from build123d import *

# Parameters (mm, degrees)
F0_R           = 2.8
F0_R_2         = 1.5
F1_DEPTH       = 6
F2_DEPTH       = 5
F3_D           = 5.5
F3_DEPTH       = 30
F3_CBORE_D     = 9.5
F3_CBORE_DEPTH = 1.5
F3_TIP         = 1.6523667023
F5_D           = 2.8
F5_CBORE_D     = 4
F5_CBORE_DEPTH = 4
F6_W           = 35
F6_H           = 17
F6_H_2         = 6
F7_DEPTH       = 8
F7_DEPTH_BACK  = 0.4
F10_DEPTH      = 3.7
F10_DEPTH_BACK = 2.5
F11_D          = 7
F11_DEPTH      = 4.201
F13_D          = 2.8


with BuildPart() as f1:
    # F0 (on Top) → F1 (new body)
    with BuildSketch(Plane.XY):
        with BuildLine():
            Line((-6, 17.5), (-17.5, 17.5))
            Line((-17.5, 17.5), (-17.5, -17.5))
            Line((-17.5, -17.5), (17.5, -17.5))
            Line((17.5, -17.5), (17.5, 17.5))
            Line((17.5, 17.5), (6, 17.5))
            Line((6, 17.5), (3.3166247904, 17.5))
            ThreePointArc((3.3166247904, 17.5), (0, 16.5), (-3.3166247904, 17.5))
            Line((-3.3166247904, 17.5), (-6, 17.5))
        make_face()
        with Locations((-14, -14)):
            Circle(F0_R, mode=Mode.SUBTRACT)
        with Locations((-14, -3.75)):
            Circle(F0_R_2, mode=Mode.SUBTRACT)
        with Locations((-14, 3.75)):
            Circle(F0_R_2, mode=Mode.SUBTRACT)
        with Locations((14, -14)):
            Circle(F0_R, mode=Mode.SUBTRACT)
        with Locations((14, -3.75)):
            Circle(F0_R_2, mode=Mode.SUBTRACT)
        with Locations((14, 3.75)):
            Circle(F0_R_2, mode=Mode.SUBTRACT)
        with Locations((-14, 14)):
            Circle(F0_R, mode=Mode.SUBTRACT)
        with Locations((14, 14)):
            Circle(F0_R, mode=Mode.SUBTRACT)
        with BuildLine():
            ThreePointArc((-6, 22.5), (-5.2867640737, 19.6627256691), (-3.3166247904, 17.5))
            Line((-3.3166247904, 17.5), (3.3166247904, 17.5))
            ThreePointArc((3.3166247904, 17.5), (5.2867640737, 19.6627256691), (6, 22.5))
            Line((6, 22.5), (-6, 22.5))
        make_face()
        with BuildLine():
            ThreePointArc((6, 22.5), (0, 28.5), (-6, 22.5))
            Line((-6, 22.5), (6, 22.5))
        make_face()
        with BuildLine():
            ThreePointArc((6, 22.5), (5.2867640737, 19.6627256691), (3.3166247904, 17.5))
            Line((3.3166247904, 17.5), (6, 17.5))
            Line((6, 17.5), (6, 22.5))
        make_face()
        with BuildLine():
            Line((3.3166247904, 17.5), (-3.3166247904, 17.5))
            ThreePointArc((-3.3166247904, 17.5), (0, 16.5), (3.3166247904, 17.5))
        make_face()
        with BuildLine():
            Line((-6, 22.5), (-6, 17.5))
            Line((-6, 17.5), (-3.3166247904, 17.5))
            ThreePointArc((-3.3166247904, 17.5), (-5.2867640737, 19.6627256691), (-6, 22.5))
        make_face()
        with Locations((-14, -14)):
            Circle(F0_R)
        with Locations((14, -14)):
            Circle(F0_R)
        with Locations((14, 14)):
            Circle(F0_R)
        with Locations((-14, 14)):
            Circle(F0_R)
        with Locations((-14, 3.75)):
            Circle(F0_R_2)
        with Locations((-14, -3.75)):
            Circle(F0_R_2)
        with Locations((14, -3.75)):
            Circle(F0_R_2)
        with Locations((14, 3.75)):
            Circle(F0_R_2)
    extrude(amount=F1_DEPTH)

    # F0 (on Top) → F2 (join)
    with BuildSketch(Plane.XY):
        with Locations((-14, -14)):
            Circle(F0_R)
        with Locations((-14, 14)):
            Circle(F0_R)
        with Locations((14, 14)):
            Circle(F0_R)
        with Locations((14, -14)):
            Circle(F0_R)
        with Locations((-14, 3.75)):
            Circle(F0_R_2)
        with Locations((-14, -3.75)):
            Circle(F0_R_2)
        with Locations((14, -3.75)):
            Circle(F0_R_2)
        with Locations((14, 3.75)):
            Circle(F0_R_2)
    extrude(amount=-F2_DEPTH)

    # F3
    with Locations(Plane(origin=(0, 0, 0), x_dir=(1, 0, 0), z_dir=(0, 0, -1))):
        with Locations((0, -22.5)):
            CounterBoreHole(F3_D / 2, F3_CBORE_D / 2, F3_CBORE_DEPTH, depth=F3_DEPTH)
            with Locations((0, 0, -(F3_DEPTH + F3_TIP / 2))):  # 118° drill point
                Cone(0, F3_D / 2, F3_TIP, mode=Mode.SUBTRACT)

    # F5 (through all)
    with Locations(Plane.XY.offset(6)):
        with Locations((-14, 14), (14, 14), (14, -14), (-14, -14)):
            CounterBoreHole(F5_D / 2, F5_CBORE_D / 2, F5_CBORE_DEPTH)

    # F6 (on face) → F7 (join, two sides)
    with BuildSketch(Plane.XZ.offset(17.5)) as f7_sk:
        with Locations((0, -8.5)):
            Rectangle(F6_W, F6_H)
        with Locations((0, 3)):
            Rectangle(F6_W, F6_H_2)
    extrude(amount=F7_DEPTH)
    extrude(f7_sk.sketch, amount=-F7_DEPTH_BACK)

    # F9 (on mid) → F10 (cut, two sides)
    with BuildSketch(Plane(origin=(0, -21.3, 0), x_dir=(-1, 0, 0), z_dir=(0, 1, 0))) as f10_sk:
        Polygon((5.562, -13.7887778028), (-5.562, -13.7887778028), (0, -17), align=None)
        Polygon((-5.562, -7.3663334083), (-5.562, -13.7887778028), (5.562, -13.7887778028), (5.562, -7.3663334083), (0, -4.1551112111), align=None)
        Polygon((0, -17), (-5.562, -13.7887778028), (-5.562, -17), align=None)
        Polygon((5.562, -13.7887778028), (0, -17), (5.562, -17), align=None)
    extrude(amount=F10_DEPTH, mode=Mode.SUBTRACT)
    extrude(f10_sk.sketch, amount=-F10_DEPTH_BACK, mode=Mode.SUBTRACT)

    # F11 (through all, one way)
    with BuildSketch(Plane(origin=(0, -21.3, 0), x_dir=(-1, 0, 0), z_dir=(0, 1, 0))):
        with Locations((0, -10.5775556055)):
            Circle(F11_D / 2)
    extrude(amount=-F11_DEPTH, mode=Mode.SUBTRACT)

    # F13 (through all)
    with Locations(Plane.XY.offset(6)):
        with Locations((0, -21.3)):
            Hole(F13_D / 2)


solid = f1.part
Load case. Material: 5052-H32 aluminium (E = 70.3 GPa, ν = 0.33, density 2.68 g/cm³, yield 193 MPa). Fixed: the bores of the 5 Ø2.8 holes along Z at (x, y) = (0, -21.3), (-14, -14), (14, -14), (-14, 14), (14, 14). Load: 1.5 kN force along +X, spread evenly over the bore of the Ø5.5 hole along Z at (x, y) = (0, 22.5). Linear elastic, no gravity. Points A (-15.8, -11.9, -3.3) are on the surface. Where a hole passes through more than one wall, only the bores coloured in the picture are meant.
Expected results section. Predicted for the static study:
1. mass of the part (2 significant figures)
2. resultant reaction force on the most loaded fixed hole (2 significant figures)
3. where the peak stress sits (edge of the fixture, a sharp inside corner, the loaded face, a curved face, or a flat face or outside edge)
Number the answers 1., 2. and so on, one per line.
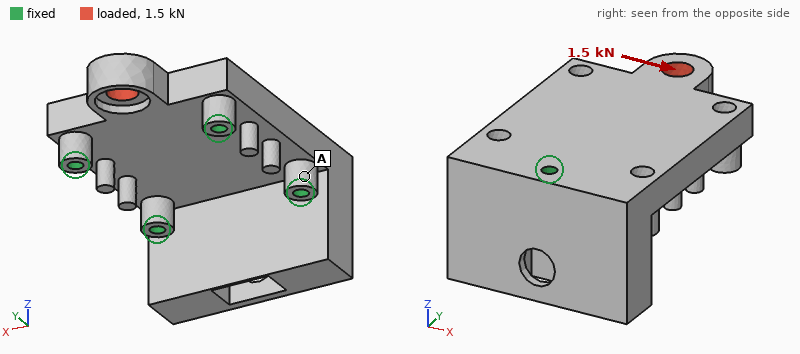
1. 37 g
2. 780 N
3. edge of the fixture
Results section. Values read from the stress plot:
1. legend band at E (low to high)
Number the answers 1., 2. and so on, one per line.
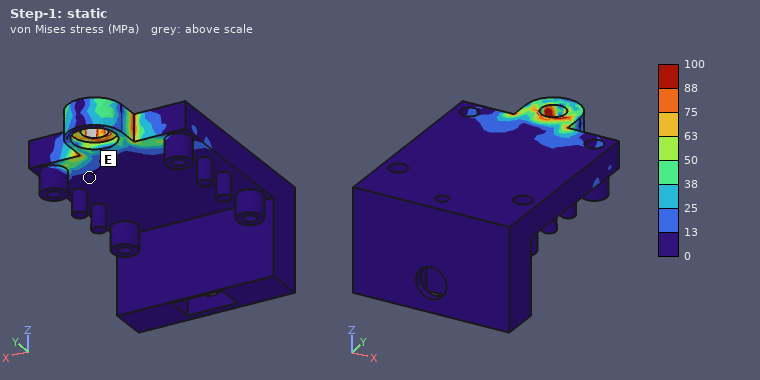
1. 0 to 13 MPa
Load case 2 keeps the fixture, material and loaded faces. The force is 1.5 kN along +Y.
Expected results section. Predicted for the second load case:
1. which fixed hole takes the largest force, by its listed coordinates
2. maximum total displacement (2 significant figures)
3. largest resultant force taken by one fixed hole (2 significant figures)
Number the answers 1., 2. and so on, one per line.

1. (0, -21.3)
2. 17 µm
3. 350 N
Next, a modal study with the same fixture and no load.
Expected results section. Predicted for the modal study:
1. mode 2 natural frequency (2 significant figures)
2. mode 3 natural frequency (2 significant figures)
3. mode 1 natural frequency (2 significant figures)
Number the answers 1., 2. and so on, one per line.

1. 15 kHz
2. 16 kHz
3. 15 kHz
